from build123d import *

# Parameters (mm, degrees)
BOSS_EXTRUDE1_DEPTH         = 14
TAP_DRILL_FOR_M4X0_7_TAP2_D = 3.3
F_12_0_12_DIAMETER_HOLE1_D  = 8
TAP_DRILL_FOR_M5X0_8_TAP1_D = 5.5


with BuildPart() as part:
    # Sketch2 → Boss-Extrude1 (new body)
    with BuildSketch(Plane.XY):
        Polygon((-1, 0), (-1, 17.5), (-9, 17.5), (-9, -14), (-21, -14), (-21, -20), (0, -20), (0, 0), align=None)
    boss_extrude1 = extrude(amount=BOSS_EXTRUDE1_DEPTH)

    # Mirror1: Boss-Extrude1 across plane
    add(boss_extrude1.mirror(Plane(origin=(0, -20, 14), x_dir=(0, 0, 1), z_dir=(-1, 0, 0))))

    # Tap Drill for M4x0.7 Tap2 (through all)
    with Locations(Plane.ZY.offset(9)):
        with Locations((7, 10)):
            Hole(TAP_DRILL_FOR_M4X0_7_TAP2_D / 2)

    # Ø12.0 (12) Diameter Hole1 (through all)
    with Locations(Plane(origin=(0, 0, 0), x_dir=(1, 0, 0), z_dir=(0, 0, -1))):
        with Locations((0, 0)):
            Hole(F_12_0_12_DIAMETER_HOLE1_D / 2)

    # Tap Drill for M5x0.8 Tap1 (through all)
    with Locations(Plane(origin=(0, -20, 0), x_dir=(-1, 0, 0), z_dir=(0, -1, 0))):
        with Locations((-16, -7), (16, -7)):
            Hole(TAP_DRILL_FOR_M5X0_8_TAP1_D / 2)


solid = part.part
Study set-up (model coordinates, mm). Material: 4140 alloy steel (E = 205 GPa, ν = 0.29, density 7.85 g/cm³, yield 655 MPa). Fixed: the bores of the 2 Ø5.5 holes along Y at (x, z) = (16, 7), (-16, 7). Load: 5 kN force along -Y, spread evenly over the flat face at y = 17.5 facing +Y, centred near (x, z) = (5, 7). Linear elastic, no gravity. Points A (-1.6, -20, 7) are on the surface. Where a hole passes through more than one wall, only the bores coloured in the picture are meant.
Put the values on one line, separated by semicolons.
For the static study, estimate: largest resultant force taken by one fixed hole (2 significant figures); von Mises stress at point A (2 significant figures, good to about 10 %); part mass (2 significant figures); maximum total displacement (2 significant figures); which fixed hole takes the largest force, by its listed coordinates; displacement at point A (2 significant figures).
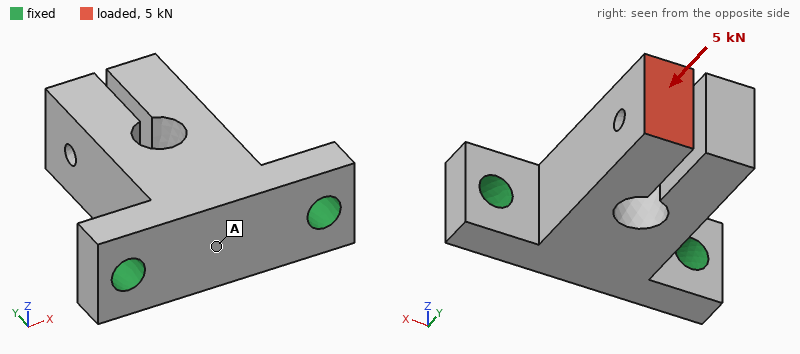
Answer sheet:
3.7 kN; 27 MPa; 78 g; 27 µm; (16, 7); 6.0 µm
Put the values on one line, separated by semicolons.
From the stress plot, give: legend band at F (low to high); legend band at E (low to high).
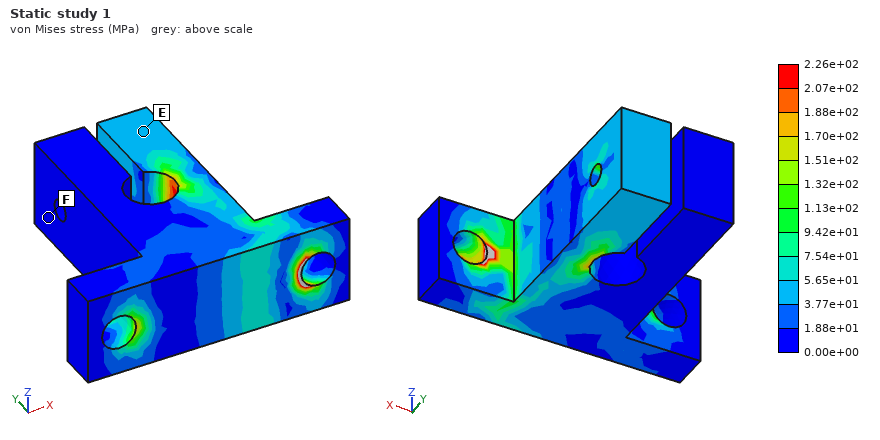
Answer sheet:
0.00e+00 to 1.88e+01 MPa; 3.77e+01 to 5.65e+01 MPa
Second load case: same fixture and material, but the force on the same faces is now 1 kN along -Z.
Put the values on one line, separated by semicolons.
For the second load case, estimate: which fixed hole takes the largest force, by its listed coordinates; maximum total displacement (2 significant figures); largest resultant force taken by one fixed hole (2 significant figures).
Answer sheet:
(16, 7); 0.10 mm; 650 N
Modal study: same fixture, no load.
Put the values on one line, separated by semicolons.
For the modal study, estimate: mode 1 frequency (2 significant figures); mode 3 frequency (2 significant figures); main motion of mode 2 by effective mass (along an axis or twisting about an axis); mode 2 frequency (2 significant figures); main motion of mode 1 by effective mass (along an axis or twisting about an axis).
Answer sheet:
4100 Hz; 6700 Hz; along X; 5800 Hz; along Z
